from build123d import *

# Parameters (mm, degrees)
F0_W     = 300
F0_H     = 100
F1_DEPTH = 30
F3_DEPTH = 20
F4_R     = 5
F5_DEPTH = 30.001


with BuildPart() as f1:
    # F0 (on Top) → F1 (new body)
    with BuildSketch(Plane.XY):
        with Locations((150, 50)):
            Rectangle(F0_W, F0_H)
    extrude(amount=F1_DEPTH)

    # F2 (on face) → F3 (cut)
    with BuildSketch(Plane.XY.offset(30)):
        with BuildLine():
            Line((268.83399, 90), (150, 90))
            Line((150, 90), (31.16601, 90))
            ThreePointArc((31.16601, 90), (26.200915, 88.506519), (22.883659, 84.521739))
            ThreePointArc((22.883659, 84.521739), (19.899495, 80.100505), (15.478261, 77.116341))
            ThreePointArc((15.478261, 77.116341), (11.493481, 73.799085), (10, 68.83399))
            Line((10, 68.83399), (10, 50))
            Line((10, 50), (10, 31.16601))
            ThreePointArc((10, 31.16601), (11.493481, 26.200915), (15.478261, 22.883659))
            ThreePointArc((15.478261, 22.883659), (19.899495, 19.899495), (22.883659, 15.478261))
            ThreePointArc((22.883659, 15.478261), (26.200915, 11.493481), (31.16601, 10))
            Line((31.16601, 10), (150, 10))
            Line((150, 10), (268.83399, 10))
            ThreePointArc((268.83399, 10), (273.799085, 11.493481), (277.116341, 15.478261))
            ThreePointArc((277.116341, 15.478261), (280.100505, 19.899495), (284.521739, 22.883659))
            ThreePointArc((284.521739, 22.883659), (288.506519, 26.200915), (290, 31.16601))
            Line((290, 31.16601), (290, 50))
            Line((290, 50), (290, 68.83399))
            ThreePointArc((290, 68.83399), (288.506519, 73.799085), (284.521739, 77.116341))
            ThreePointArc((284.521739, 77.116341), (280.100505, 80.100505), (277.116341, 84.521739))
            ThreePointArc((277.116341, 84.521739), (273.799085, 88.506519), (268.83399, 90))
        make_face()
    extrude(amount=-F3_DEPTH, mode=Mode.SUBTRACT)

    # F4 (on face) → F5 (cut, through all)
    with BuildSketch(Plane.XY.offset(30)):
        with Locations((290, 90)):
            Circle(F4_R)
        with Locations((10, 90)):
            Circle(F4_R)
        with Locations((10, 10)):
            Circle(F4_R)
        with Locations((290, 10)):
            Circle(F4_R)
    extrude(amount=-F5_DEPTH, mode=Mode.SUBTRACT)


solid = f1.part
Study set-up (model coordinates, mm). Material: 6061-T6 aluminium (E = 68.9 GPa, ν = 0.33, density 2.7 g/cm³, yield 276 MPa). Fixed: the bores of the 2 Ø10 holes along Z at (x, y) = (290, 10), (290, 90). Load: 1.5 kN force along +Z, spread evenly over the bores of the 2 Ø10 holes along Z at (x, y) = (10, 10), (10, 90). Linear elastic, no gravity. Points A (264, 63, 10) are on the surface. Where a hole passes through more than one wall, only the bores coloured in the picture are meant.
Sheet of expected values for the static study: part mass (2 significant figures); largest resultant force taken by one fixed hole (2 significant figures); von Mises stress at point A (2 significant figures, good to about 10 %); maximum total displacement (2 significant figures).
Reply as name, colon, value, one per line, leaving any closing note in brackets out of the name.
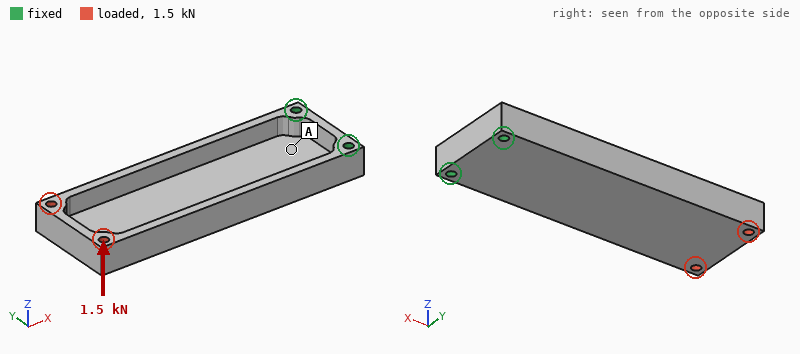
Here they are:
part mass: 1.2 kg
largest resultant force taken by one fixed hole: 2.3 kN
von Mises stress at point A: 15 MPa
maximum total displacement: 2.0 mm
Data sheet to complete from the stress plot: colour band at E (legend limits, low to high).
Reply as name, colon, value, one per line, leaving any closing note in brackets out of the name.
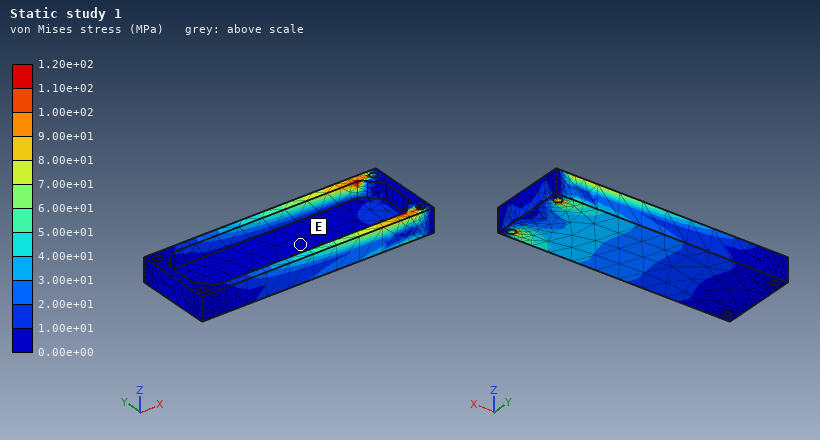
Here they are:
colour band at E: 0.00e+00 to 1.00e+01 MPa
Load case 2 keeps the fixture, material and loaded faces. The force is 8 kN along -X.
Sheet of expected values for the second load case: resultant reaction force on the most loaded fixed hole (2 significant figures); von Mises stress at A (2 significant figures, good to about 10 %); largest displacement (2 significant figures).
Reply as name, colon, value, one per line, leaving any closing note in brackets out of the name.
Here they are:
resultant reaction force on the most loaded fixed hole: 4.0 kN
von Mises stress at A: 4.7 MPa
largest displacement: 0.31 mm
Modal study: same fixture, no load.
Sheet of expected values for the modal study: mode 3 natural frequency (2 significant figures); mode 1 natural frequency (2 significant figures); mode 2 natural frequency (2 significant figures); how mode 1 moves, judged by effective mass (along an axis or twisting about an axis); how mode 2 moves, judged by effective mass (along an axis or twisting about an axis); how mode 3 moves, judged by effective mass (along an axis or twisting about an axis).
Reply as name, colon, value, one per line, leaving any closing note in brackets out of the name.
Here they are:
mode 3 natural frequency: 1000 Hz
mode 1 natural frequency: 240 Hz
mode 2 natural frequency: 570 Hz
how mode 1 moves, judged by effective mass: along Z
how mode 2 moves, judged by effective mass: along Y
how mode 3 moves, judged by effective mass: along Y
